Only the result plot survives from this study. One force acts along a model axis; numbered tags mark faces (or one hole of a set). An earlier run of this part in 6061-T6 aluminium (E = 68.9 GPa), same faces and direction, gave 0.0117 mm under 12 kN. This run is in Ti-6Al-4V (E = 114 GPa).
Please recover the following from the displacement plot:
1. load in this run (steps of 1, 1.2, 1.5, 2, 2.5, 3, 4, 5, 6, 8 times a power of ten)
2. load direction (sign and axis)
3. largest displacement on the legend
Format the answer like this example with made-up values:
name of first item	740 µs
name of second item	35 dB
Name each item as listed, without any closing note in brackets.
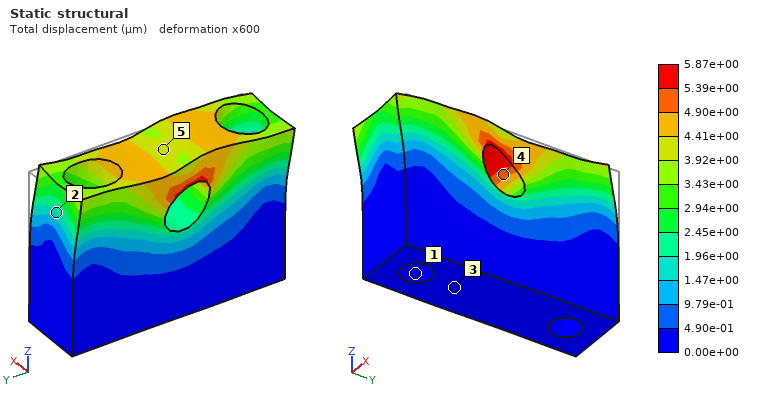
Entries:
load in this run	10 kN
load direction	-Y
largest displacement on the legend	5.87e+00 µm
